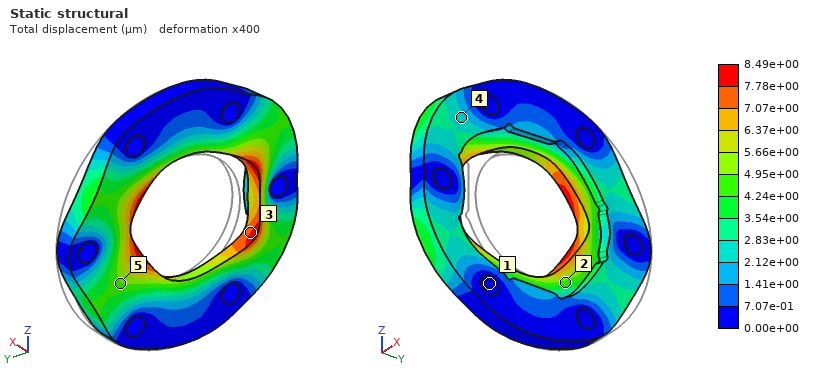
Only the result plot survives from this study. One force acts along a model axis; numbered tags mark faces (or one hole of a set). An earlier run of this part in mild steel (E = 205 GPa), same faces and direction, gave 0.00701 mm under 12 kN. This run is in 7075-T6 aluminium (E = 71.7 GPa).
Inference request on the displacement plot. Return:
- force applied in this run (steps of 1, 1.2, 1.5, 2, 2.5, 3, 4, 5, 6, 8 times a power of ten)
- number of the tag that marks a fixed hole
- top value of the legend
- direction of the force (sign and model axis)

5 kN
1
8.49e+00 µm
-Y
